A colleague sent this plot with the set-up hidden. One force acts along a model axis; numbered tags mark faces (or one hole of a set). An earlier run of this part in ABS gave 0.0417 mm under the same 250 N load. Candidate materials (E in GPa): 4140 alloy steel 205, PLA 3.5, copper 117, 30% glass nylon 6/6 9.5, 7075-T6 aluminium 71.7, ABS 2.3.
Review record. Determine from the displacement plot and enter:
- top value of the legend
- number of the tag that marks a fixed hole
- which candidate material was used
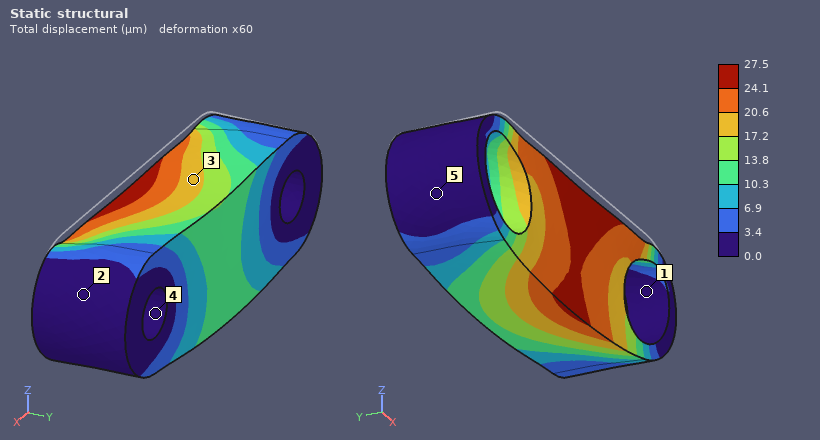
27.5 µm
4
PLA
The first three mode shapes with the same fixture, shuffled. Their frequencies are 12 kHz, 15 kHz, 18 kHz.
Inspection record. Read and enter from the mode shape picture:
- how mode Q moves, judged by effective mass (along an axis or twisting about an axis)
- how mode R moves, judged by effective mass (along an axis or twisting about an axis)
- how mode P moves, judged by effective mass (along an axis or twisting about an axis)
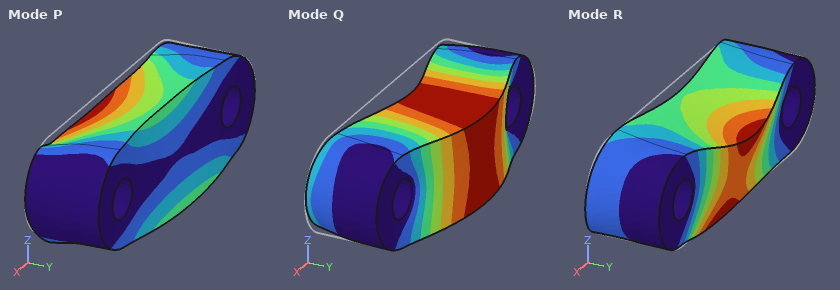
along Y
along Z
along Z
